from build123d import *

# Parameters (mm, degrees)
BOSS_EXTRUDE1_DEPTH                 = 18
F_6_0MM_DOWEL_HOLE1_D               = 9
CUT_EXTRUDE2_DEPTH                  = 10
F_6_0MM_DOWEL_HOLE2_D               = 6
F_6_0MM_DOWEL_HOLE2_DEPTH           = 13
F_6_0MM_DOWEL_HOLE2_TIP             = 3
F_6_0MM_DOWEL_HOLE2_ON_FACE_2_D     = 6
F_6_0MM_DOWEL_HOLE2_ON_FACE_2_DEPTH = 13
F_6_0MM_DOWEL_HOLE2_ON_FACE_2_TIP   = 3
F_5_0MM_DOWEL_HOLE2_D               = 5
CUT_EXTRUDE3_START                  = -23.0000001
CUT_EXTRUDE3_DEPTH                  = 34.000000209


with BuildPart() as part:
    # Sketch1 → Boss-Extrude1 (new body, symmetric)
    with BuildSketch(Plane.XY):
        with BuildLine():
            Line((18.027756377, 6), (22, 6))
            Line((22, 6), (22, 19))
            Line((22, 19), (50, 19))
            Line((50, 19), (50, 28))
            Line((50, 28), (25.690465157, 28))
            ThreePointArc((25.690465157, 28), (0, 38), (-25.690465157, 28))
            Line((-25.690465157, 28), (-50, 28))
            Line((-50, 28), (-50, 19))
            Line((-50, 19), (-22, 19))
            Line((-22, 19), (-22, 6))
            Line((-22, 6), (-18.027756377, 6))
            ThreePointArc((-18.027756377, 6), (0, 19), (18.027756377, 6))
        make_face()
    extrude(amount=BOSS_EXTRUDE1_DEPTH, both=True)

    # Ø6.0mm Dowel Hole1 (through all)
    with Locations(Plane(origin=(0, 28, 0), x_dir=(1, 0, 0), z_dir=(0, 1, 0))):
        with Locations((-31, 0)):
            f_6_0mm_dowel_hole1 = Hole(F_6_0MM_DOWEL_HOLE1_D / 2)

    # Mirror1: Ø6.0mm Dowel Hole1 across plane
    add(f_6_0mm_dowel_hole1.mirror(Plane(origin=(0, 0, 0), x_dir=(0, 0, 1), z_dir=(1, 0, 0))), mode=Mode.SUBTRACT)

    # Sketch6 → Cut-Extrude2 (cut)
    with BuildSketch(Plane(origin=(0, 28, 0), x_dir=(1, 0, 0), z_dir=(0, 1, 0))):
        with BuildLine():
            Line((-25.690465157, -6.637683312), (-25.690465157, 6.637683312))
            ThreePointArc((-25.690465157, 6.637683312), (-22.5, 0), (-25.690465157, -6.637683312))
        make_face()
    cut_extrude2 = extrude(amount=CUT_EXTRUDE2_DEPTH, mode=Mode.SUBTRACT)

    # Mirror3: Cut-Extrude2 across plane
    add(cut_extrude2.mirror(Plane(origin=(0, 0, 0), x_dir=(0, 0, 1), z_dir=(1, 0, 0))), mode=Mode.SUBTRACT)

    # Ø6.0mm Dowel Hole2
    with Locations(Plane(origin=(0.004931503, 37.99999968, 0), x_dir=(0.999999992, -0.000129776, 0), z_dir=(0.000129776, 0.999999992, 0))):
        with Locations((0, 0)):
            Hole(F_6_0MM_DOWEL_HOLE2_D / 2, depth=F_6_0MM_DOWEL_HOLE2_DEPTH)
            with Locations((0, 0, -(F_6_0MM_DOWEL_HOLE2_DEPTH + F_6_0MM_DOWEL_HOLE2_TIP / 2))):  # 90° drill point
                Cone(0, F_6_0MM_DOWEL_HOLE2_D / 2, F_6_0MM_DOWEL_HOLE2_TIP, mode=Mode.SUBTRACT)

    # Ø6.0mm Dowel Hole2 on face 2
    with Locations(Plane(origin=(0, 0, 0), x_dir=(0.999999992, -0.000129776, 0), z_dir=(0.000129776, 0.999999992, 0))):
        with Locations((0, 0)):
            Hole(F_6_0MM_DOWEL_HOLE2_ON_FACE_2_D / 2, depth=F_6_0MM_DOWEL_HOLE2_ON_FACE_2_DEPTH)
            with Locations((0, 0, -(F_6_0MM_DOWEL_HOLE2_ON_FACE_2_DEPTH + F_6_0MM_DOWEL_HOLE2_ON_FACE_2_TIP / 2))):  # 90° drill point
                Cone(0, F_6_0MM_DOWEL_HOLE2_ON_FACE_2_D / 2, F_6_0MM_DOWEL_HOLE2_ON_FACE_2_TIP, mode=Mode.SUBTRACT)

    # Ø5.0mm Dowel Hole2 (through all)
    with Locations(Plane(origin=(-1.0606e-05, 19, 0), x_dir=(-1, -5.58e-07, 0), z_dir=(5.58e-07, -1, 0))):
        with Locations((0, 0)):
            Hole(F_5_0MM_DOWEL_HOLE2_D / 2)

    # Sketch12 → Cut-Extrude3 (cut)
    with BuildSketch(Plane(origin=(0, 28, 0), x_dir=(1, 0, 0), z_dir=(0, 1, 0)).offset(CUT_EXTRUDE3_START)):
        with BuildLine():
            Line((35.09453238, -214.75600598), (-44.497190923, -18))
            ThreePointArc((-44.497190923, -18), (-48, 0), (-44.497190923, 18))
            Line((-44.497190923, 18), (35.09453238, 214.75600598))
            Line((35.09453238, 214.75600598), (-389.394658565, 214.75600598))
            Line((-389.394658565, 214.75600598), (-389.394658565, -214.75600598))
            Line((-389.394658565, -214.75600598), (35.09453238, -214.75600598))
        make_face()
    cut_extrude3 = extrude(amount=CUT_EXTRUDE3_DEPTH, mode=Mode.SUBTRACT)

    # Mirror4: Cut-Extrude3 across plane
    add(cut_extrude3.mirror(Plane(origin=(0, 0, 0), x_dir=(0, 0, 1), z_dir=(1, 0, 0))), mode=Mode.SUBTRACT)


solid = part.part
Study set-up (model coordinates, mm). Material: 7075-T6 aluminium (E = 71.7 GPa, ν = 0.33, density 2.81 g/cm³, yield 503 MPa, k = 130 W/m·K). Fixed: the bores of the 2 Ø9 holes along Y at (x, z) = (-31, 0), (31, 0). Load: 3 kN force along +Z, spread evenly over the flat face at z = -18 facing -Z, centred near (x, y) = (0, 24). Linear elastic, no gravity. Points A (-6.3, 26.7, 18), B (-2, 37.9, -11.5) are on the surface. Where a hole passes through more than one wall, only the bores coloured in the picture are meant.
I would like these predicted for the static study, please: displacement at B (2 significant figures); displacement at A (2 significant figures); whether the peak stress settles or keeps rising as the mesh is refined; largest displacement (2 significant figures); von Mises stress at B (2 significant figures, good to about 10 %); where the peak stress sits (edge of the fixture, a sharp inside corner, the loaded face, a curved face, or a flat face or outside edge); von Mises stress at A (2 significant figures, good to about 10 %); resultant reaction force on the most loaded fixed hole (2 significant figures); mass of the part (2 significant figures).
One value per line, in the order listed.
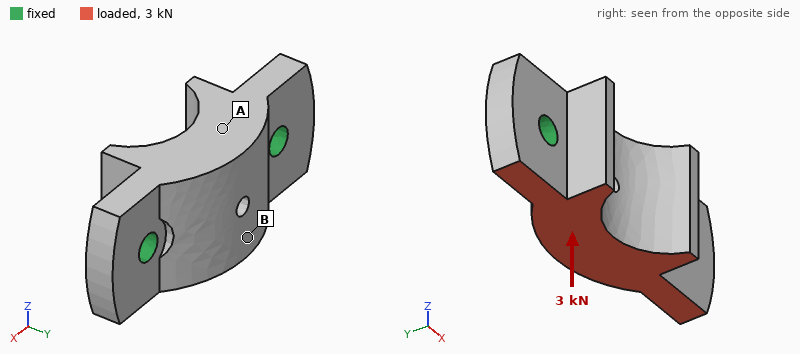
4.1 µm
2.8 µm
keeps rising
4.4 µm
1.7 MPa
edge of the fixture
3.8 MPa
1.5 kN
140 g
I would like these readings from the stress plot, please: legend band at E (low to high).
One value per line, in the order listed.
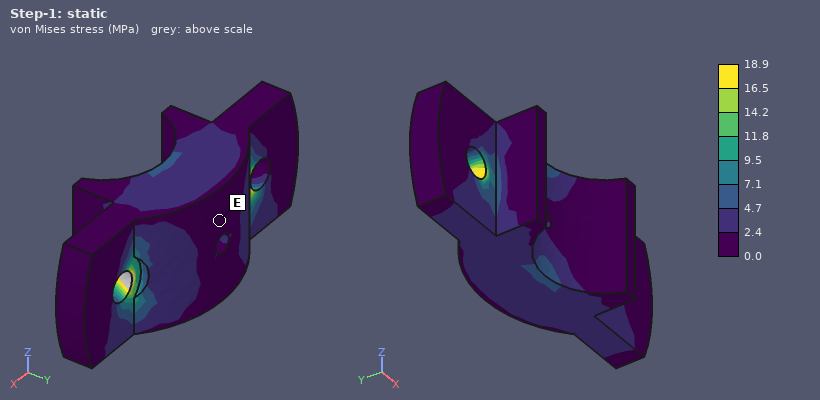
0.0 to 2.4 MPa
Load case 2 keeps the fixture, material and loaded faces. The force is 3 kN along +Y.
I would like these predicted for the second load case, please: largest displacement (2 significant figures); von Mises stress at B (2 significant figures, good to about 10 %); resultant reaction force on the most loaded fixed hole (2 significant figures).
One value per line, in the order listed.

26 µm
9.2 MPa
1.6 kN
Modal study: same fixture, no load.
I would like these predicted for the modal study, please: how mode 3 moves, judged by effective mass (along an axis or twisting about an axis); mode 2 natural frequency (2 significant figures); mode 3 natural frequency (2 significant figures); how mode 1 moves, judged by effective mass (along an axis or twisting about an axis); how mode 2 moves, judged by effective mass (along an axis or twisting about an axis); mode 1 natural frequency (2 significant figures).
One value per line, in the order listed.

along Z
11 kHz
15 kHz
twisting about X
along Y
9000 Hz
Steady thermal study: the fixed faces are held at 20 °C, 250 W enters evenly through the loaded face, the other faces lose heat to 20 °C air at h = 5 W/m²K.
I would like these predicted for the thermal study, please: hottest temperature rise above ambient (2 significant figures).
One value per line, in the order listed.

54 K
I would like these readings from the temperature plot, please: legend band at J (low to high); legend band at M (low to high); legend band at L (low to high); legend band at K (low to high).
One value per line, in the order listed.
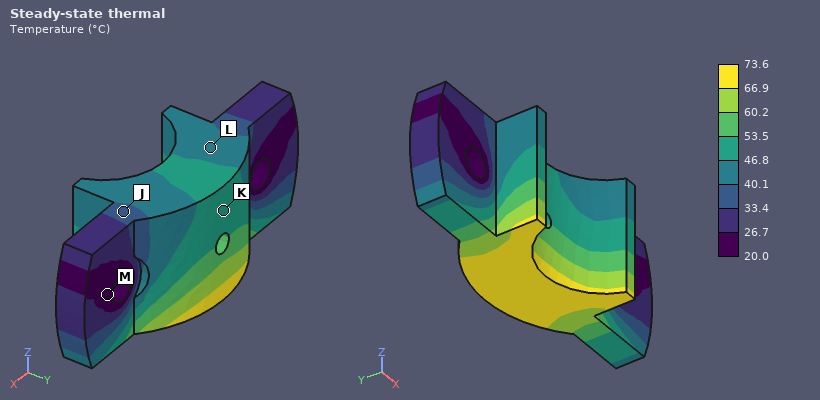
33.4 to 40.1 °C
20.0 to 26.7 °C
40.1 to 46.8 °C
46.8 to 53.5 °C
